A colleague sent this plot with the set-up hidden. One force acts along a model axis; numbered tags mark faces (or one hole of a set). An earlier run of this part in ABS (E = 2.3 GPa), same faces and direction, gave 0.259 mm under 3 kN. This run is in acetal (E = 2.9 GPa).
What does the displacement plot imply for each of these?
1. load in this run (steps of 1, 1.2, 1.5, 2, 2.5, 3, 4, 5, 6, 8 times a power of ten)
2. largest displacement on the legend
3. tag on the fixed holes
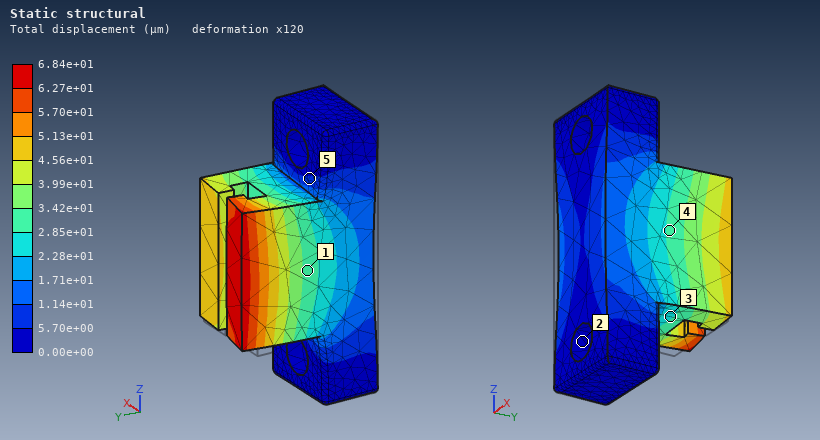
1 kN
6.84e+01 µm
2
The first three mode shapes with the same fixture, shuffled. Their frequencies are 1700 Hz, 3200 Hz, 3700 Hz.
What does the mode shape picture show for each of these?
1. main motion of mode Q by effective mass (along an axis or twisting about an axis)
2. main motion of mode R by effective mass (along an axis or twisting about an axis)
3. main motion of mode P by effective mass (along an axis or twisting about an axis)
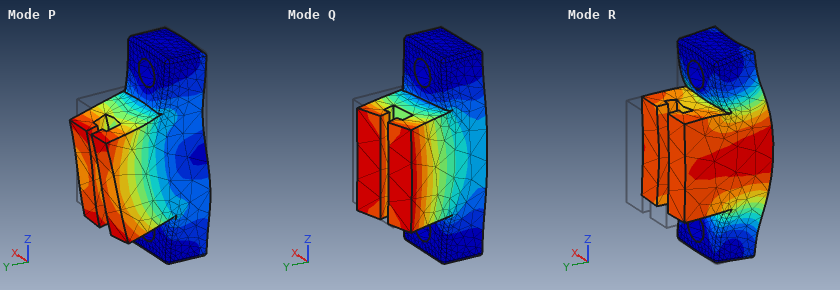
along X
along Y
along Z
